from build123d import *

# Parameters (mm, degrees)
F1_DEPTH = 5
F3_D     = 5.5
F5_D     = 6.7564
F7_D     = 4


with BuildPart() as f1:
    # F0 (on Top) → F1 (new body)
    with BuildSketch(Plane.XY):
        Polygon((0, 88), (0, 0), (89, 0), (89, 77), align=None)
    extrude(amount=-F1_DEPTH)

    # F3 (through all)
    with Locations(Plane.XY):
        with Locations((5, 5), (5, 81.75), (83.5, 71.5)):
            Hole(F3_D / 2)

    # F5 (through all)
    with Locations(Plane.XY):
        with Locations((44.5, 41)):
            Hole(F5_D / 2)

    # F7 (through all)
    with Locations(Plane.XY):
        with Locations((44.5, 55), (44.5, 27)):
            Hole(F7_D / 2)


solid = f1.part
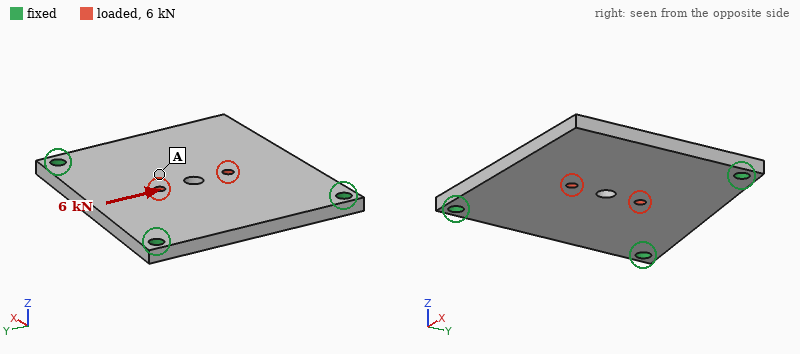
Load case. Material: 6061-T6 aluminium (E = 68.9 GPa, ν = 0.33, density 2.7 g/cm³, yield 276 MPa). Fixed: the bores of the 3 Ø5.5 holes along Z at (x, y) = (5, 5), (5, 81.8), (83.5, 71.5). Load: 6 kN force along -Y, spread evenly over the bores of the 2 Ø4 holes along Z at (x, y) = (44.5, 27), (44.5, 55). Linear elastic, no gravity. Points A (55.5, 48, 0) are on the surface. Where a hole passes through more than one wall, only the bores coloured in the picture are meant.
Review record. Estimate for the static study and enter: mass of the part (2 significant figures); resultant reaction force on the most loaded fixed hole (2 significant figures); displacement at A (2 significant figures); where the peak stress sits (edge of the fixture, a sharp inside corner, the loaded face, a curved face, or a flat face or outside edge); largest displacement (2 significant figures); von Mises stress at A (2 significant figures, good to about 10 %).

97 g
2.4 kN
17 µm
edge of the fixture
22 µm
14 MPa
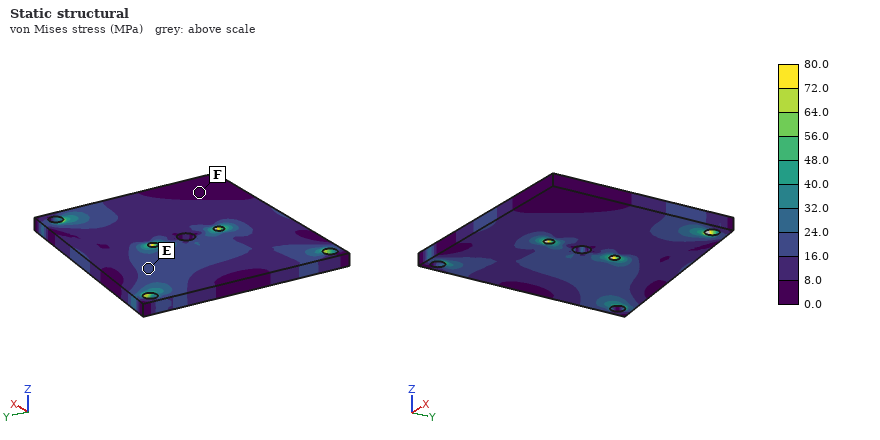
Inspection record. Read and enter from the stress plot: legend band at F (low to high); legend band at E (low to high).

0.0 to 8.0 MPa
16.0 to 24.0 MPa
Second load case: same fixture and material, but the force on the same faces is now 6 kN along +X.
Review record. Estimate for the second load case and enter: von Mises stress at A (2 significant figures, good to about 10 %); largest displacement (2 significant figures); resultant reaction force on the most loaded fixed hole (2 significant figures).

8.3 MPa
19 µm
2.3 kN
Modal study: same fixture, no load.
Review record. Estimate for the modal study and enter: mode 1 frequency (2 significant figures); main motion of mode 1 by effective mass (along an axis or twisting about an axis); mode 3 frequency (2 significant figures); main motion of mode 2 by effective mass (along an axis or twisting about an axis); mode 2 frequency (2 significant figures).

1300 Hz
along Z
4500 Hz
along Z
3100 Hz
